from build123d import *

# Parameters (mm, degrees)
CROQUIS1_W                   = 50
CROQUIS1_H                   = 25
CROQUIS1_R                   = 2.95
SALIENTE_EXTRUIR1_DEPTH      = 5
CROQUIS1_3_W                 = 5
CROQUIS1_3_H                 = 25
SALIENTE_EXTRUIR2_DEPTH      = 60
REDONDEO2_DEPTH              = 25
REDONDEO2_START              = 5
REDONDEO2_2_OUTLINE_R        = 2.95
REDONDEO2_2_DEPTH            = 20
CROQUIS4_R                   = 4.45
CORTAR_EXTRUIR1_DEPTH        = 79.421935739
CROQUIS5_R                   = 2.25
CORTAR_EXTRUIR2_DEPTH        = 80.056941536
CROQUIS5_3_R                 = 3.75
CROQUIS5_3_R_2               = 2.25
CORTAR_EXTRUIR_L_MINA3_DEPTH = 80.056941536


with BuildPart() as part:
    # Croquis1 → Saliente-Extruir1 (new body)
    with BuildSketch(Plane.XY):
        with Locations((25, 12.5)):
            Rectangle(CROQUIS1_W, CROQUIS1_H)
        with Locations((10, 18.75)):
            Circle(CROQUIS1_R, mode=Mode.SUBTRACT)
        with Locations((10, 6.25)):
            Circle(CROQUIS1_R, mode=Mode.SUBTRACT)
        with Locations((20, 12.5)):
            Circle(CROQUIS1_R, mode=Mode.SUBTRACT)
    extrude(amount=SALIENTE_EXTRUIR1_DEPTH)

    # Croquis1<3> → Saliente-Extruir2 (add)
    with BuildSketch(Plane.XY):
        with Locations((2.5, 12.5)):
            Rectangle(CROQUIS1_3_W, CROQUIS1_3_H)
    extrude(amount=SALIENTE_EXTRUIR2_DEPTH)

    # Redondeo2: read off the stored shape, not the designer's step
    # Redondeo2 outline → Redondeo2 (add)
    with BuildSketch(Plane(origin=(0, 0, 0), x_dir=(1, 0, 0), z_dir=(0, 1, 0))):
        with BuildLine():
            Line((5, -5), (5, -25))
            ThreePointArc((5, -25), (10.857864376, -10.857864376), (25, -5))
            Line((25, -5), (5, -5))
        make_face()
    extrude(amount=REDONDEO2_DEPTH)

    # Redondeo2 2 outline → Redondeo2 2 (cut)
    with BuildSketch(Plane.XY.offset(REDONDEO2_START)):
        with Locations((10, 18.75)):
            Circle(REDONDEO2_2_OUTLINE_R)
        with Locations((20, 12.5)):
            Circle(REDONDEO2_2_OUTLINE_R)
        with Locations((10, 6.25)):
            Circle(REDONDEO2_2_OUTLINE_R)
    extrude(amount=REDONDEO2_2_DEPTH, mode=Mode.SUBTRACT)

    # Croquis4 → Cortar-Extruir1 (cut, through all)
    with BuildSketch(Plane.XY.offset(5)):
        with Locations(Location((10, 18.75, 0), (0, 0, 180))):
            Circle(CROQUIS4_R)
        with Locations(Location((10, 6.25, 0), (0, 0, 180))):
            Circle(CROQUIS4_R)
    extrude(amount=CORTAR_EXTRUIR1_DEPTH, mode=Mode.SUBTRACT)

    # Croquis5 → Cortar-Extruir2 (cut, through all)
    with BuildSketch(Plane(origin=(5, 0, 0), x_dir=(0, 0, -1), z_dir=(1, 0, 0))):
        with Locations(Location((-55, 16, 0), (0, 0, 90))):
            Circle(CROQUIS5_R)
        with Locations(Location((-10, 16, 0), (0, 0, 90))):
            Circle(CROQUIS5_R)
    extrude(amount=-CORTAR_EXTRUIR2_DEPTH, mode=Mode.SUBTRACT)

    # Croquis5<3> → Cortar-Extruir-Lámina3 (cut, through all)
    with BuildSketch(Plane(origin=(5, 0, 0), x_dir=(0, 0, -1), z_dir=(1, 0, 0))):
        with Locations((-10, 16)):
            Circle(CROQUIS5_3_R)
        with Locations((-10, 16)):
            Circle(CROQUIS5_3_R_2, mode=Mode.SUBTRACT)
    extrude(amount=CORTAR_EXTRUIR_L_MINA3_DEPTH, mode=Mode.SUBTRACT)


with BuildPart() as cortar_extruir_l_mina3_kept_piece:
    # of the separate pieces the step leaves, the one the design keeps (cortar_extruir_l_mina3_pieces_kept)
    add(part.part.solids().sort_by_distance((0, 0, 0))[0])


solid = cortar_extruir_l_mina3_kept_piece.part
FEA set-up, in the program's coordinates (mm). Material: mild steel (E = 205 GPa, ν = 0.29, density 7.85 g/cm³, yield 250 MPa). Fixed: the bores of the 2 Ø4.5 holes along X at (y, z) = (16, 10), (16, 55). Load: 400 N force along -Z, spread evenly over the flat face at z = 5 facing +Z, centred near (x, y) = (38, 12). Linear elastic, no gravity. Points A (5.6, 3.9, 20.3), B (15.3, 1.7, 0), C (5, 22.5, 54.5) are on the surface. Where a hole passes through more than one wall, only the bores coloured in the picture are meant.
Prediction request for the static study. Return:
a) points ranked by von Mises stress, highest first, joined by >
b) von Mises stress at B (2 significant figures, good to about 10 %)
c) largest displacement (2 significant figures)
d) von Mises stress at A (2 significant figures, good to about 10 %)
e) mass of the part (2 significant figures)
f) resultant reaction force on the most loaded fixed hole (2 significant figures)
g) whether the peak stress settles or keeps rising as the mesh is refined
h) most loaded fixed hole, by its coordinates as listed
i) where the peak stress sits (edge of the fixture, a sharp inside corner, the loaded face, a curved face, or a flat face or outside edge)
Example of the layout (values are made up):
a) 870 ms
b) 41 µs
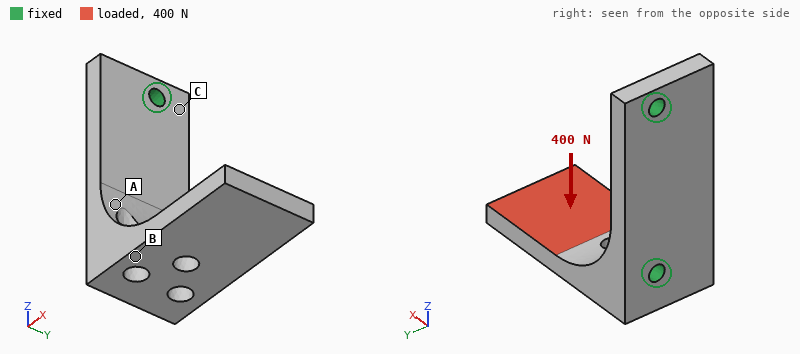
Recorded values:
a) B > A > C
b) 58 MPa
c) 0.11 mm
d) 27 MPa
e) 110 g
f) 280 N
g) keeps rising
h) (16, 10)
i) edge of the fixture
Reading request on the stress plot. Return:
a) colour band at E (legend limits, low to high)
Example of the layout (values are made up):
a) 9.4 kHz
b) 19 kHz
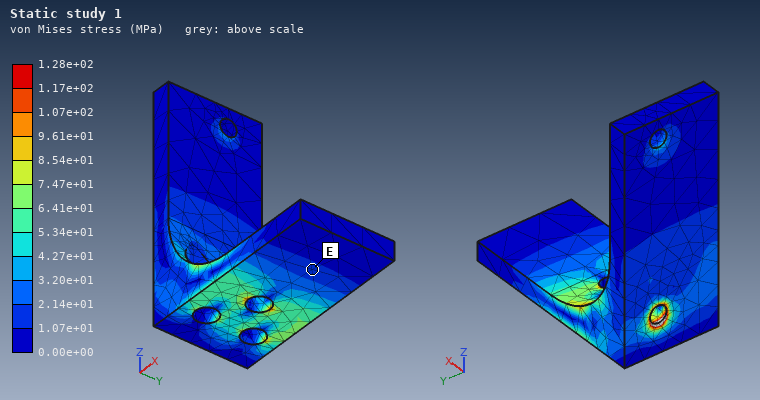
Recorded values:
a) 1.07e+01 to 2.14e+01 MPa
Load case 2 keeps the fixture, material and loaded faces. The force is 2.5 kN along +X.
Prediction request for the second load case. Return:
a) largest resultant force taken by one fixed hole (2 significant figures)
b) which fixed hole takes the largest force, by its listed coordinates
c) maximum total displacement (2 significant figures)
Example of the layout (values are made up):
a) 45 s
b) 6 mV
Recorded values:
a) 2.6 kN
b) (16, 10)
c) 45 µm
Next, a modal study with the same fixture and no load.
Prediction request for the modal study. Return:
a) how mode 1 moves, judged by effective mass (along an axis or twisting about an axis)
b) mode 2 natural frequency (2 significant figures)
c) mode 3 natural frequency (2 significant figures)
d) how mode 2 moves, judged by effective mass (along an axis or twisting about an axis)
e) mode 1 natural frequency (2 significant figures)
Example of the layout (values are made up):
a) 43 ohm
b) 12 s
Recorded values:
a) along Z
b) 3100 Hz
c) 7900 Hz
d) along Y
e) 2300 Hz
